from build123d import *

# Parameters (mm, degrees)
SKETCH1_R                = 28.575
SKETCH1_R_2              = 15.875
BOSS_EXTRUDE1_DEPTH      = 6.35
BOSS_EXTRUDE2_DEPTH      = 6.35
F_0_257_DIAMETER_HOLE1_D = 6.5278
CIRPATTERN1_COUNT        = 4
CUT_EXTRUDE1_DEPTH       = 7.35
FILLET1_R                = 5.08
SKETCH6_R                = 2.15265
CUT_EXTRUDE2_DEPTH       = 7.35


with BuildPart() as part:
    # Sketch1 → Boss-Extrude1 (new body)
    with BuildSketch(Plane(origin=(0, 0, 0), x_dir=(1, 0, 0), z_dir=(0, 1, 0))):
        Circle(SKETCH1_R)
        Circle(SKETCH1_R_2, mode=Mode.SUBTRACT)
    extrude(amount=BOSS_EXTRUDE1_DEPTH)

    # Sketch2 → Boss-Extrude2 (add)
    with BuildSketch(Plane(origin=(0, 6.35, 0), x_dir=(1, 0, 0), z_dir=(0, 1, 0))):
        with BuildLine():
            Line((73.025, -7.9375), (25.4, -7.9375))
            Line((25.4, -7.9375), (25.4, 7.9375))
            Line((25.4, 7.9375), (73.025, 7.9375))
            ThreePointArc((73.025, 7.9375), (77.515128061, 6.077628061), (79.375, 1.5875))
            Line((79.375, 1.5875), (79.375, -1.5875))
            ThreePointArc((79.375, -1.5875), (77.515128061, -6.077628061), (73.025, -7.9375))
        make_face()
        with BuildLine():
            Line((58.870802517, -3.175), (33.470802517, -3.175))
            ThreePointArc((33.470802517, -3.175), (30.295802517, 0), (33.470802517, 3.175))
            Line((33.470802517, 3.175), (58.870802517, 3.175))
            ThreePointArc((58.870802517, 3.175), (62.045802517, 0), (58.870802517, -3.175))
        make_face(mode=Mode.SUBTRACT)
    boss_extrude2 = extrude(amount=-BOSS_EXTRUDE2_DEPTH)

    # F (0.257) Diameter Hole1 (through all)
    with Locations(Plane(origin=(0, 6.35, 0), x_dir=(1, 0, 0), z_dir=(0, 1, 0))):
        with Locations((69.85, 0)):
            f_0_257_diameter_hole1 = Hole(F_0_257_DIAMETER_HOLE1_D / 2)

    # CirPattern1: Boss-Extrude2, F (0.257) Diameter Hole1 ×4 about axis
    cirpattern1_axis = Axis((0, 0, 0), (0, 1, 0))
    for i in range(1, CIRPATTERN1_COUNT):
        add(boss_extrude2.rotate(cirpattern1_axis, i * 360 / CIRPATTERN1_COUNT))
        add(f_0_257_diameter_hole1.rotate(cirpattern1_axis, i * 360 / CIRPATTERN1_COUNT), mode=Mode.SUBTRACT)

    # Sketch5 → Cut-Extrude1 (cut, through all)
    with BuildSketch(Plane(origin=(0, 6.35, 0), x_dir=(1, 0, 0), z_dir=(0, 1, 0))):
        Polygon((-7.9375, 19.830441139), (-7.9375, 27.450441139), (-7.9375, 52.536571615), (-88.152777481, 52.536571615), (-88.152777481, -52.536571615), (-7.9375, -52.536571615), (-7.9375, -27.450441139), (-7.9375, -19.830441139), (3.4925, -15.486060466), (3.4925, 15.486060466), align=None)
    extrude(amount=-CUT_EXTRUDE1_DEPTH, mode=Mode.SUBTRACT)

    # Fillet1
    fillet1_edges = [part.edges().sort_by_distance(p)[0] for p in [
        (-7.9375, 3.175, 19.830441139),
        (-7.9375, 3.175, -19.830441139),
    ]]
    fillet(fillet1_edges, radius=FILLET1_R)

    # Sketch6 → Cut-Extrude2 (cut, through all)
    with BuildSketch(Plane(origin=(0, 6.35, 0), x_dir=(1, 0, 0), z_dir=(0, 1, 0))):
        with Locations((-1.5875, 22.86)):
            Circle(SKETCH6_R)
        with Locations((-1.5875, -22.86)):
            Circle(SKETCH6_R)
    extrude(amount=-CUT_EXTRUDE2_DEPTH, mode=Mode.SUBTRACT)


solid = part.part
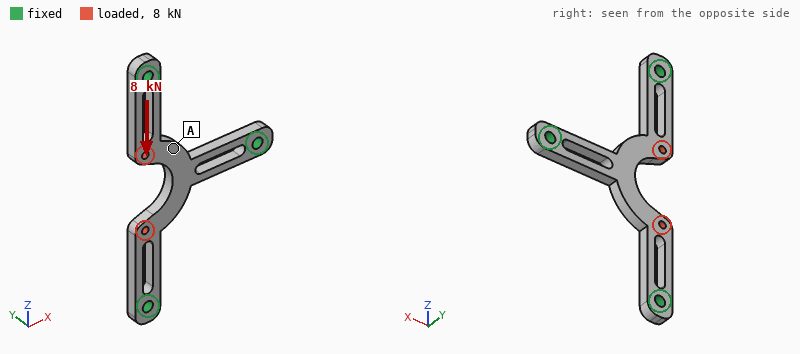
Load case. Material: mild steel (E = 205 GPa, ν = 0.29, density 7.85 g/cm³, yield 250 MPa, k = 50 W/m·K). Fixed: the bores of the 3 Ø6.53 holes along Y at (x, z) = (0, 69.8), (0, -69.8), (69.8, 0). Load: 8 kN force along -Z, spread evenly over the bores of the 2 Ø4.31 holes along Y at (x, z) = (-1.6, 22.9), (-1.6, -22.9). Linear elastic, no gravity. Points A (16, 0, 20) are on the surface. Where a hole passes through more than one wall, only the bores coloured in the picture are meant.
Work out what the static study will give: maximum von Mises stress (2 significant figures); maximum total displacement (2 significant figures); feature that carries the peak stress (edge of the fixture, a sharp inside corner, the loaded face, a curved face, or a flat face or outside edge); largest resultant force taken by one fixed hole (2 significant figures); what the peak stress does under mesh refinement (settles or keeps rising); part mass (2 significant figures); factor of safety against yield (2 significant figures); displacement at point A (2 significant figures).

130 MPa
18 µm
a curved face
4.0 kN
settles
140 g
2.0
10 µm
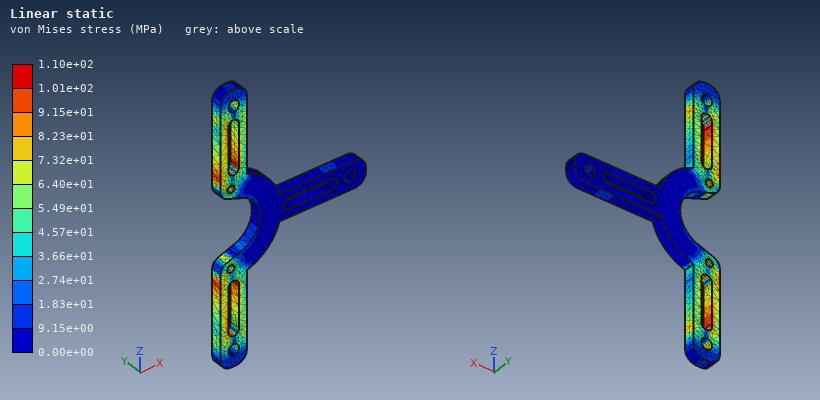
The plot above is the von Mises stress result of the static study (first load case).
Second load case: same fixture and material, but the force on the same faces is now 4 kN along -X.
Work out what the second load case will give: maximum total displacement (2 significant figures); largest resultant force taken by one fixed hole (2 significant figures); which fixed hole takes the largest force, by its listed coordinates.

23 µm
3.7 kN
(69.8, 0)
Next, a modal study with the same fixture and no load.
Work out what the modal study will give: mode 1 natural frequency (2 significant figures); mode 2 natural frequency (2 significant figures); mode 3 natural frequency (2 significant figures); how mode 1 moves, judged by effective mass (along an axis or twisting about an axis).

1900 Hz
3900 Hz
5200 Hz
along Y
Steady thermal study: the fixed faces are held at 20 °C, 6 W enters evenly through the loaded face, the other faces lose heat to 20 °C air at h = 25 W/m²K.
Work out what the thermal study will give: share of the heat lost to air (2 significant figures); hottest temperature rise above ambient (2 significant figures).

38 %
23 K
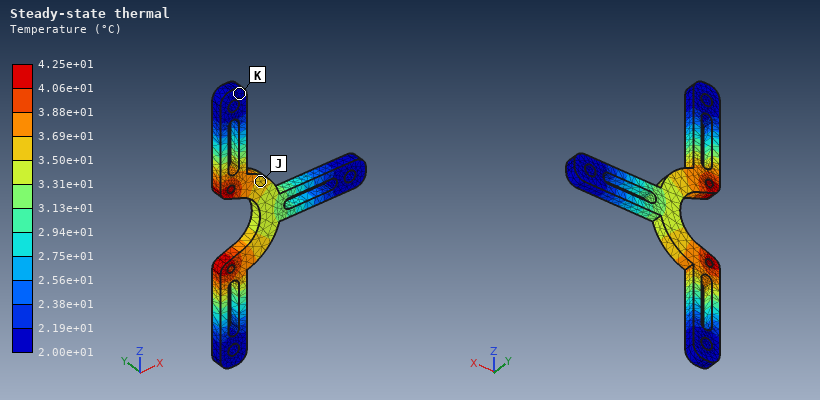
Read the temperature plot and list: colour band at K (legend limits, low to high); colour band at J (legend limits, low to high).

2.00e+01 to 2.19e+01 °C
3.50e+01 to 3.69e+01 °C
